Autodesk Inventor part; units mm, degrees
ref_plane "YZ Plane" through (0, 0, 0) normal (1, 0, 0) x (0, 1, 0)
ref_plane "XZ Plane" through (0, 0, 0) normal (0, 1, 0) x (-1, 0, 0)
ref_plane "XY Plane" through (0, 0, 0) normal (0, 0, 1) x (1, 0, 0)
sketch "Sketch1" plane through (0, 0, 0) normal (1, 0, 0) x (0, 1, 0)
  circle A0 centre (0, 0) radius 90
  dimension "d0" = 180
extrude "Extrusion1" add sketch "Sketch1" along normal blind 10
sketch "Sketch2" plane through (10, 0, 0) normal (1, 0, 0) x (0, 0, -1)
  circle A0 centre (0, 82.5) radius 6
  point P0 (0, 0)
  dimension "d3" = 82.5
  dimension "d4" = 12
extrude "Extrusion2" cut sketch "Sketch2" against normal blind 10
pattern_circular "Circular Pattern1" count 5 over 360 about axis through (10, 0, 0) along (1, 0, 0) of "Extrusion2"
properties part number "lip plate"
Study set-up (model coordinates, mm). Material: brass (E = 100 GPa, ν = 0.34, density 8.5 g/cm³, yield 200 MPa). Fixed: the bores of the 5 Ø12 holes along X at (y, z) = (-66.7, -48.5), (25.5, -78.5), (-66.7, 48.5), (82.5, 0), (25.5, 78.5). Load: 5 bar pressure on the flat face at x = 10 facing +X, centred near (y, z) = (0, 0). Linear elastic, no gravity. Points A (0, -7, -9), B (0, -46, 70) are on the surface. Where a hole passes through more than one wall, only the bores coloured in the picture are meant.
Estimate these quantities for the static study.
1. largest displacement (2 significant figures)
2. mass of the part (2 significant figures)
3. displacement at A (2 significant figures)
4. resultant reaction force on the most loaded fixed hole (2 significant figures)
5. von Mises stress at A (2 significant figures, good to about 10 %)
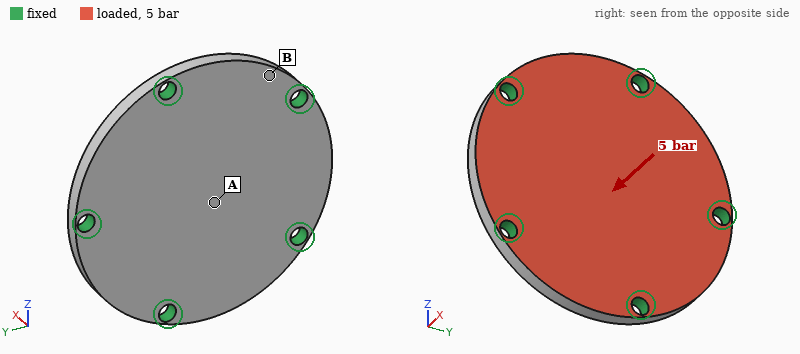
55 µm
2.1 kg
53 µm
2.5 kN
18 MPa
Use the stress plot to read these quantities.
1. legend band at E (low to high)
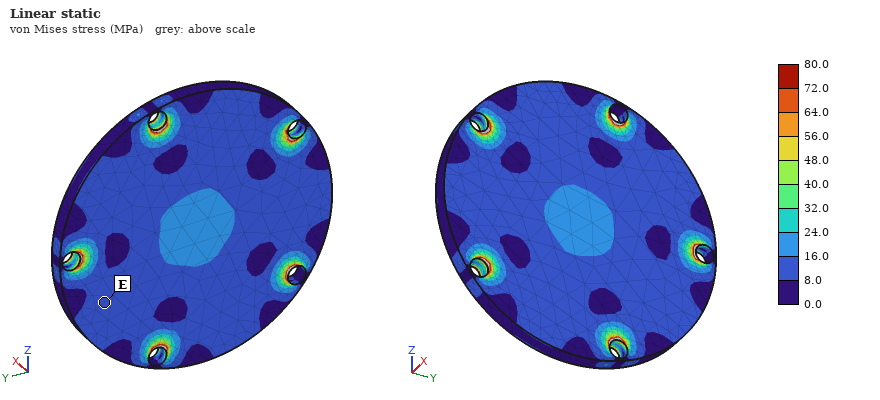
8.0 to 16.0 MPa
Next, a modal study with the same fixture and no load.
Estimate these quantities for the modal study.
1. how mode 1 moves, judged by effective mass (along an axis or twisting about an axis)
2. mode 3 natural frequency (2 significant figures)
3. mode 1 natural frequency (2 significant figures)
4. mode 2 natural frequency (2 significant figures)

along X
3600 Hz
2000 Hz
3600 Hz
